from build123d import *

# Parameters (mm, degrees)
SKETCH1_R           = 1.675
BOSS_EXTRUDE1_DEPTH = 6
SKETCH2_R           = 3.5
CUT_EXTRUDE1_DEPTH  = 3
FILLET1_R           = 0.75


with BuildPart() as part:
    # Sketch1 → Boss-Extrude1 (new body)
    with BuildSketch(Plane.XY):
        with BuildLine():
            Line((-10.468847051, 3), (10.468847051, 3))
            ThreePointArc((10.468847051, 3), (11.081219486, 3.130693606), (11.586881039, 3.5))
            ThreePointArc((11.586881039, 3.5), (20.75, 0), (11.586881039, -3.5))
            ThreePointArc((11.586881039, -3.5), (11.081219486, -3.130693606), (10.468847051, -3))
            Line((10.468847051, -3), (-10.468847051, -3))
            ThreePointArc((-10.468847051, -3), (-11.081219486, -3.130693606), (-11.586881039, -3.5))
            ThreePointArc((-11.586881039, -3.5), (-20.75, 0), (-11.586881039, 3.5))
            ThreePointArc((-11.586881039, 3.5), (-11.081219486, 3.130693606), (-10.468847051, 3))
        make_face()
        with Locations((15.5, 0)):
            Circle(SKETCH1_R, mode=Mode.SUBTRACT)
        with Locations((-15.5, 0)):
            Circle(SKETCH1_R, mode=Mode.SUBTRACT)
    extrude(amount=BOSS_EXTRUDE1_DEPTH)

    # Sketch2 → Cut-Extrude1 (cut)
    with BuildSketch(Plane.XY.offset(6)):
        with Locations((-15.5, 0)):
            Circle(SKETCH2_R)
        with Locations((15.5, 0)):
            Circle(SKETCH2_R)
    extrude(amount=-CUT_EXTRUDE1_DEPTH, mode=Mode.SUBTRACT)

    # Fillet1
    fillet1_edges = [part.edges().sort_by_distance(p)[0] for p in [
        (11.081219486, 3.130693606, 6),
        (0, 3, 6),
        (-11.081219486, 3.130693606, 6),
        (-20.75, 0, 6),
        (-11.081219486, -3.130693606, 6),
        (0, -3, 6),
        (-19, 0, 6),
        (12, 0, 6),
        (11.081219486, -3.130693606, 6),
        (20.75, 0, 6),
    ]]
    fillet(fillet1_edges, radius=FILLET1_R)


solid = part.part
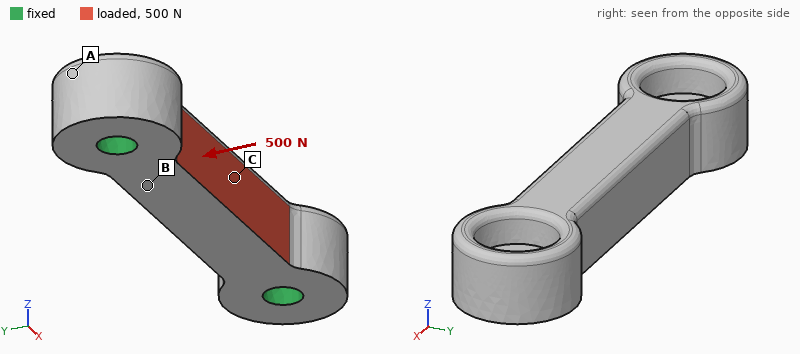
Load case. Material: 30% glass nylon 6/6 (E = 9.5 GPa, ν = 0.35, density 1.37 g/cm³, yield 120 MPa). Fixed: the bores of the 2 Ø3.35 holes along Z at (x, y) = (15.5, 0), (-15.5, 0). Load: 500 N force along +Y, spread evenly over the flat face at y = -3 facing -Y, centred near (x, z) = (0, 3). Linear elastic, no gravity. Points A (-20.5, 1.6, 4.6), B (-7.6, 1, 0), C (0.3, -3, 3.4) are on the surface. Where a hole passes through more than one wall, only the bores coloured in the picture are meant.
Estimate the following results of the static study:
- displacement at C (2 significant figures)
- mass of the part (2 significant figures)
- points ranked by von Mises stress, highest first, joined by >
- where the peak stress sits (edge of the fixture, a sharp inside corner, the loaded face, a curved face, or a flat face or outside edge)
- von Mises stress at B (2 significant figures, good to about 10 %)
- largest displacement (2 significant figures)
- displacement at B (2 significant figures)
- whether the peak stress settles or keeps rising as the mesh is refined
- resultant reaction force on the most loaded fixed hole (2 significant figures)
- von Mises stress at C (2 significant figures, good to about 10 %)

80 µm
2.1 g
C > B > A
edge of the fixture
17 MPa
82 µm
48 µm
keeps rising
250 N
26 MPa
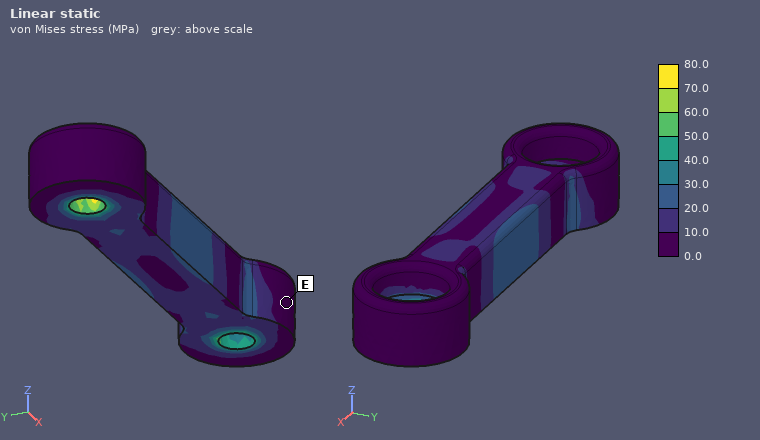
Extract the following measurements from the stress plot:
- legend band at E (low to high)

0.0 to 10.0 MPa
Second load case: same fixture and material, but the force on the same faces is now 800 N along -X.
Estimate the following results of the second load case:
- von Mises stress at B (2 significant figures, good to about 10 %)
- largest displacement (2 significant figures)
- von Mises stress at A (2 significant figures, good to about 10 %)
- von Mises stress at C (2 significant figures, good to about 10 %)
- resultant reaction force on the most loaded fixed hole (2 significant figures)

13 MPa
24 µm
2.4 MPa
13 MPa
410 N
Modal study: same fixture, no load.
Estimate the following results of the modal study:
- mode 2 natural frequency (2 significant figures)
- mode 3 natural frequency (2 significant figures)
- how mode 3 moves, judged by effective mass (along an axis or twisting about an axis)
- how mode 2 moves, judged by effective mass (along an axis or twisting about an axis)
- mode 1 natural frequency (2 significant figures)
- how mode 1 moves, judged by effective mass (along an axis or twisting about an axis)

13 kHz
22 kHz
twisting about X
along Y
12 kHz
along Z
